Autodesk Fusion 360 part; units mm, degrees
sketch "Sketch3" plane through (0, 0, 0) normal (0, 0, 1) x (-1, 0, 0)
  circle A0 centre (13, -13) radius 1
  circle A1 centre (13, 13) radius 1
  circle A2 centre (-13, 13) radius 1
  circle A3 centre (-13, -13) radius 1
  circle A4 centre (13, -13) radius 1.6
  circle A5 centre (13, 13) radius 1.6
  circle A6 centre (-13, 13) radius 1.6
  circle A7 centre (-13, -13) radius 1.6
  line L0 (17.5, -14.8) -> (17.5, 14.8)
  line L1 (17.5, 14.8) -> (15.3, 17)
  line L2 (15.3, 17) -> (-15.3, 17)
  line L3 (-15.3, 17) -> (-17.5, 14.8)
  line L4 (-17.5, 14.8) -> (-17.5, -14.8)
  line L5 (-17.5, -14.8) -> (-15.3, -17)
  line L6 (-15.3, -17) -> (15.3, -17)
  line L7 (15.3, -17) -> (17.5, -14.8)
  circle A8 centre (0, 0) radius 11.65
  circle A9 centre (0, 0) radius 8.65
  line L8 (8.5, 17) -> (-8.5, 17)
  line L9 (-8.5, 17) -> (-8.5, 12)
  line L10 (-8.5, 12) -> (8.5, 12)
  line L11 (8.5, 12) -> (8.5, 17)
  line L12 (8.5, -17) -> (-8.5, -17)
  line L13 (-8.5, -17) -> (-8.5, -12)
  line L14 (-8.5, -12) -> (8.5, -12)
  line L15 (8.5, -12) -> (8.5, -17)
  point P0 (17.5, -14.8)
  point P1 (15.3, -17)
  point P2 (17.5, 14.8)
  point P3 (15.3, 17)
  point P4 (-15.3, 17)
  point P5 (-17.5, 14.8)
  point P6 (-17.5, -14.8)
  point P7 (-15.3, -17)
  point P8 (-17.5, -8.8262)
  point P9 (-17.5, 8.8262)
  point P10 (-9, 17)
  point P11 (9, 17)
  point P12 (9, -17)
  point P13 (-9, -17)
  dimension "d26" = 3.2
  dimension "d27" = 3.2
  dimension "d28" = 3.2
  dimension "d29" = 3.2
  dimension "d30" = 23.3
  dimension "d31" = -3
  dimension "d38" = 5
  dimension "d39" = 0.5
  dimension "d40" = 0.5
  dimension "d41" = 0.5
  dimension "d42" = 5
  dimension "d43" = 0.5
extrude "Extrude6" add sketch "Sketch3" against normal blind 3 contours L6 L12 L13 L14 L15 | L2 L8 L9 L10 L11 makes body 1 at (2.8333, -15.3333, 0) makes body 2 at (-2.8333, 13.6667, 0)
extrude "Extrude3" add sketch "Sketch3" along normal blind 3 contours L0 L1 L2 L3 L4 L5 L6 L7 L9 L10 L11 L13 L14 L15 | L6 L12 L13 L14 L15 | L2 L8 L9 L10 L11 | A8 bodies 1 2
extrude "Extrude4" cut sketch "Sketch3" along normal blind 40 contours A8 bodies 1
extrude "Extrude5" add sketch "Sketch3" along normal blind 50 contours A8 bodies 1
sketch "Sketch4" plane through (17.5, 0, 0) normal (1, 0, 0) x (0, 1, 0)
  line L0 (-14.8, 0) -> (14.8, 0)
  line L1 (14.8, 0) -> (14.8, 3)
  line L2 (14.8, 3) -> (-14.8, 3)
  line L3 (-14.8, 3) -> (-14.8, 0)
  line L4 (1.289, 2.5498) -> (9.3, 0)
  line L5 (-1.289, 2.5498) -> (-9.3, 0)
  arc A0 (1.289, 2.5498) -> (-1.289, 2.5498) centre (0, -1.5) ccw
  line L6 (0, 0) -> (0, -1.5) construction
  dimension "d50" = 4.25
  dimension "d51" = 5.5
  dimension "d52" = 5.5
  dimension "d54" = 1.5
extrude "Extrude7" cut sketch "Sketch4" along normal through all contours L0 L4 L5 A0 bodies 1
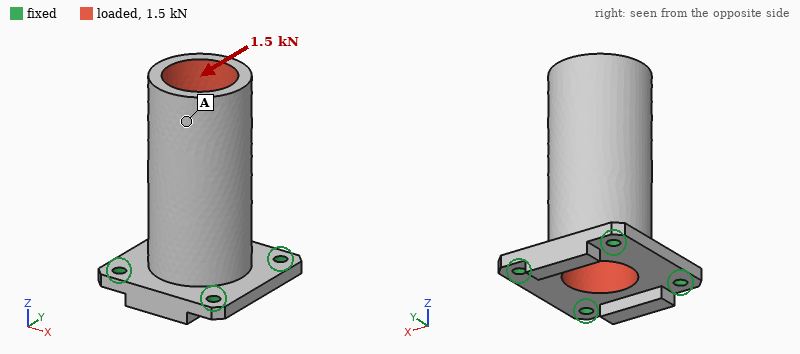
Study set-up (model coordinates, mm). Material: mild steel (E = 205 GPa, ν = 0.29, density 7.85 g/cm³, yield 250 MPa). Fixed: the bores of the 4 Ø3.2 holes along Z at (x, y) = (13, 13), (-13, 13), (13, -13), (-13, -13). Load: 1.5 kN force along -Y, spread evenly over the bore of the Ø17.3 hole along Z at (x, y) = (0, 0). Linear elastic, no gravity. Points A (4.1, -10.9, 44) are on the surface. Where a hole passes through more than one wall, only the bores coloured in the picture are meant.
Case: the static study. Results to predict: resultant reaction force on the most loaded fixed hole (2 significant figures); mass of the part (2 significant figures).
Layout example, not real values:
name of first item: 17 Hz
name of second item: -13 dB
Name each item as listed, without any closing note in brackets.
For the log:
resultant reaction force on the most loaded fixed hole: 840 N
mass of the part: 96 g
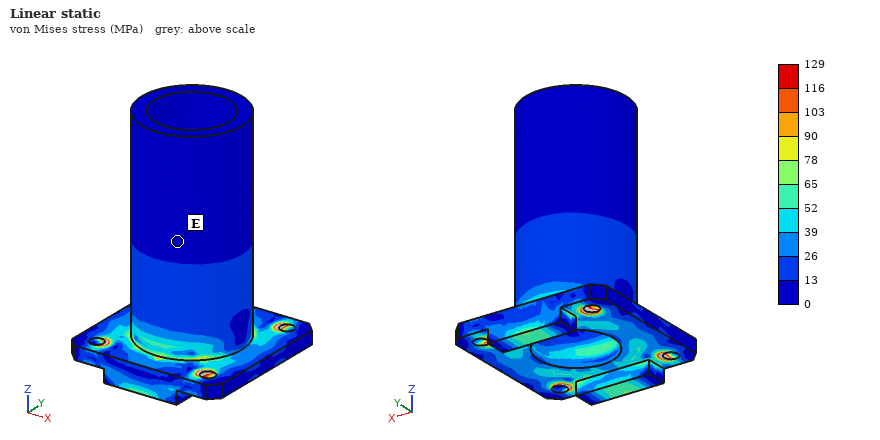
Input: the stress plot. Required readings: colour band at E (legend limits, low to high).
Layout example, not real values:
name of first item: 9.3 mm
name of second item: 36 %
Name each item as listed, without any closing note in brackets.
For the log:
colour band at E: 0 to 13 MPa
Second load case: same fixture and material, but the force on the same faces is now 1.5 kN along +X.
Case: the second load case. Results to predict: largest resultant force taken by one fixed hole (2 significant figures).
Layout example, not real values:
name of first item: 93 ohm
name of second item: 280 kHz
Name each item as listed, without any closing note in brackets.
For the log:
largest resultant force taken by one fixed hole: 900 N
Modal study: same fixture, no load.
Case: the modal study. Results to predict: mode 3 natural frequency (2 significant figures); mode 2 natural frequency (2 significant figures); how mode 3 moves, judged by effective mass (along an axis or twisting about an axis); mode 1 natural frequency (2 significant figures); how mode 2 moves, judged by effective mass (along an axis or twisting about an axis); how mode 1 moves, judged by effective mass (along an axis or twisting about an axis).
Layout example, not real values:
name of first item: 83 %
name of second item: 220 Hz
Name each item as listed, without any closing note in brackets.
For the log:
mode 3 natural frequency: 10 kHz
mode 2 natural frequency: 3900 Hz
how mode 3 moves, judged by effective mass: along Z
mode 1 natural frequency: 3600 Hz
how mode 2 moves, judged by effective mass: along Y
how mode 1 moves, judged by effective mass: along X
